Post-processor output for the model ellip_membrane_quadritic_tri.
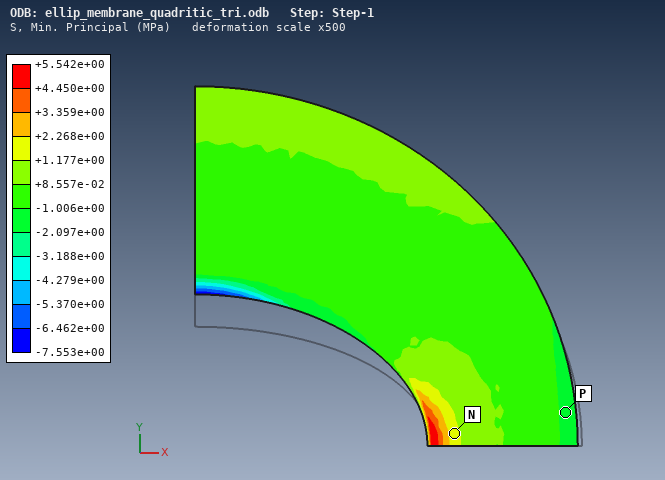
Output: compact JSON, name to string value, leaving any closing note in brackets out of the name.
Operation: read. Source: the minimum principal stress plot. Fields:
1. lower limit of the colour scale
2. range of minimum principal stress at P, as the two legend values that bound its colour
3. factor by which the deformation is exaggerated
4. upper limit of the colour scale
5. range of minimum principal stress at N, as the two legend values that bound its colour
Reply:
{"lower limit of the colour scale": "-7.553e+00 MPa", "range of minimum principal stress at P, as the two legend values that bound its colour": "-2.097e+00 to -1.006e+00 MPa", "factor by which the deformation is exaggerated": "500", "upper limit of the colour scale": "+5.542e+00 MPa", "range of minimum principal stress at N, as the two legend values that bound its colour": "+1.177e+00 to +2.268e+00 MPa"}
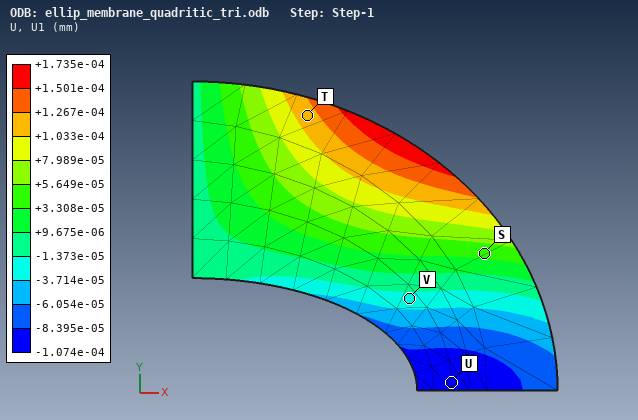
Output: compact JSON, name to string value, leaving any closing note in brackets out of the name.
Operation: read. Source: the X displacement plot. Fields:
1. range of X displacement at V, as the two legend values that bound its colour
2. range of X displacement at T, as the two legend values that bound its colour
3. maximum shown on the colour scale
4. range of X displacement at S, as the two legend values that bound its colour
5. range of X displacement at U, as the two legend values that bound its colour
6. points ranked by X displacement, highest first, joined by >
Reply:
{"range of X displacement at V, as the two legend values that bound its colour": "-3.714e-05 to -1.373e-05 mm", "range of X displacement at T, as the two legend values that bound its colour": "+1.033e-04 to +1.267e-04 mm", "maximum shown on the colour scale": "+1.735e-04 mm", "range of X displacement at S, as the two legend values that bound its colour": "+3.308e-05 to +5.649e-05 mm", "range of X displacement at U, as the two legend values that bound its colour": "-1.074e-04 to -8.395e-05 mm", "points ranked by X displacement, highest first, joined by >": "T > S > V > U"}
